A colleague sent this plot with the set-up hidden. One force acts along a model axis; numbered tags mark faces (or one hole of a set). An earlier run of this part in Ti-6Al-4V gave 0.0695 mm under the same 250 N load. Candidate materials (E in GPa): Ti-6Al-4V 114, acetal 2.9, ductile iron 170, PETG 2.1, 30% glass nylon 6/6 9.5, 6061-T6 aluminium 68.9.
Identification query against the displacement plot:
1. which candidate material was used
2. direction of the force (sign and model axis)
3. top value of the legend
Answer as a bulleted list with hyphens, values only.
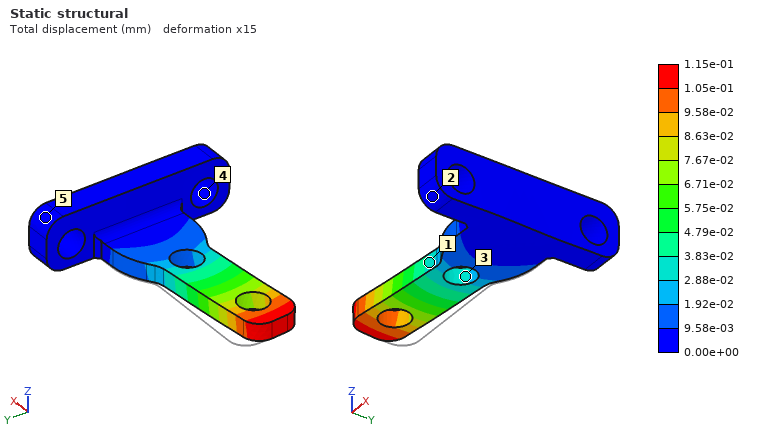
- 6061-T6 aluminium
- -Y
- 1.15e-01 mm
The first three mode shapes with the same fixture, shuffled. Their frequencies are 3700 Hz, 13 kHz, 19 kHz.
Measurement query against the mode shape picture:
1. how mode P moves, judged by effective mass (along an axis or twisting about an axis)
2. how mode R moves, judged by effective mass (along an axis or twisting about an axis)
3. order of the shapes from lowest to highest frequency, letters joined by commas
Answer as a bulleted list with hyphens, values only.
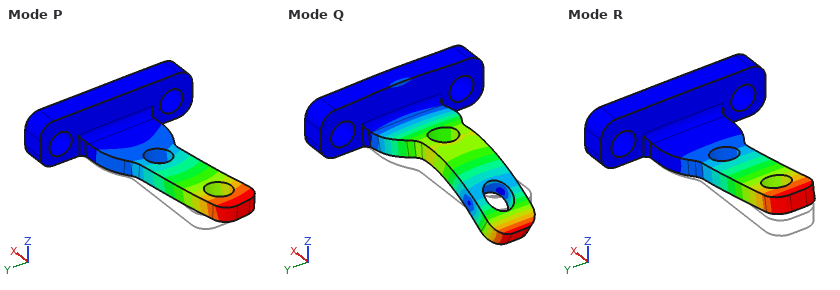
- along Y
- along Z
- R, P, Q
